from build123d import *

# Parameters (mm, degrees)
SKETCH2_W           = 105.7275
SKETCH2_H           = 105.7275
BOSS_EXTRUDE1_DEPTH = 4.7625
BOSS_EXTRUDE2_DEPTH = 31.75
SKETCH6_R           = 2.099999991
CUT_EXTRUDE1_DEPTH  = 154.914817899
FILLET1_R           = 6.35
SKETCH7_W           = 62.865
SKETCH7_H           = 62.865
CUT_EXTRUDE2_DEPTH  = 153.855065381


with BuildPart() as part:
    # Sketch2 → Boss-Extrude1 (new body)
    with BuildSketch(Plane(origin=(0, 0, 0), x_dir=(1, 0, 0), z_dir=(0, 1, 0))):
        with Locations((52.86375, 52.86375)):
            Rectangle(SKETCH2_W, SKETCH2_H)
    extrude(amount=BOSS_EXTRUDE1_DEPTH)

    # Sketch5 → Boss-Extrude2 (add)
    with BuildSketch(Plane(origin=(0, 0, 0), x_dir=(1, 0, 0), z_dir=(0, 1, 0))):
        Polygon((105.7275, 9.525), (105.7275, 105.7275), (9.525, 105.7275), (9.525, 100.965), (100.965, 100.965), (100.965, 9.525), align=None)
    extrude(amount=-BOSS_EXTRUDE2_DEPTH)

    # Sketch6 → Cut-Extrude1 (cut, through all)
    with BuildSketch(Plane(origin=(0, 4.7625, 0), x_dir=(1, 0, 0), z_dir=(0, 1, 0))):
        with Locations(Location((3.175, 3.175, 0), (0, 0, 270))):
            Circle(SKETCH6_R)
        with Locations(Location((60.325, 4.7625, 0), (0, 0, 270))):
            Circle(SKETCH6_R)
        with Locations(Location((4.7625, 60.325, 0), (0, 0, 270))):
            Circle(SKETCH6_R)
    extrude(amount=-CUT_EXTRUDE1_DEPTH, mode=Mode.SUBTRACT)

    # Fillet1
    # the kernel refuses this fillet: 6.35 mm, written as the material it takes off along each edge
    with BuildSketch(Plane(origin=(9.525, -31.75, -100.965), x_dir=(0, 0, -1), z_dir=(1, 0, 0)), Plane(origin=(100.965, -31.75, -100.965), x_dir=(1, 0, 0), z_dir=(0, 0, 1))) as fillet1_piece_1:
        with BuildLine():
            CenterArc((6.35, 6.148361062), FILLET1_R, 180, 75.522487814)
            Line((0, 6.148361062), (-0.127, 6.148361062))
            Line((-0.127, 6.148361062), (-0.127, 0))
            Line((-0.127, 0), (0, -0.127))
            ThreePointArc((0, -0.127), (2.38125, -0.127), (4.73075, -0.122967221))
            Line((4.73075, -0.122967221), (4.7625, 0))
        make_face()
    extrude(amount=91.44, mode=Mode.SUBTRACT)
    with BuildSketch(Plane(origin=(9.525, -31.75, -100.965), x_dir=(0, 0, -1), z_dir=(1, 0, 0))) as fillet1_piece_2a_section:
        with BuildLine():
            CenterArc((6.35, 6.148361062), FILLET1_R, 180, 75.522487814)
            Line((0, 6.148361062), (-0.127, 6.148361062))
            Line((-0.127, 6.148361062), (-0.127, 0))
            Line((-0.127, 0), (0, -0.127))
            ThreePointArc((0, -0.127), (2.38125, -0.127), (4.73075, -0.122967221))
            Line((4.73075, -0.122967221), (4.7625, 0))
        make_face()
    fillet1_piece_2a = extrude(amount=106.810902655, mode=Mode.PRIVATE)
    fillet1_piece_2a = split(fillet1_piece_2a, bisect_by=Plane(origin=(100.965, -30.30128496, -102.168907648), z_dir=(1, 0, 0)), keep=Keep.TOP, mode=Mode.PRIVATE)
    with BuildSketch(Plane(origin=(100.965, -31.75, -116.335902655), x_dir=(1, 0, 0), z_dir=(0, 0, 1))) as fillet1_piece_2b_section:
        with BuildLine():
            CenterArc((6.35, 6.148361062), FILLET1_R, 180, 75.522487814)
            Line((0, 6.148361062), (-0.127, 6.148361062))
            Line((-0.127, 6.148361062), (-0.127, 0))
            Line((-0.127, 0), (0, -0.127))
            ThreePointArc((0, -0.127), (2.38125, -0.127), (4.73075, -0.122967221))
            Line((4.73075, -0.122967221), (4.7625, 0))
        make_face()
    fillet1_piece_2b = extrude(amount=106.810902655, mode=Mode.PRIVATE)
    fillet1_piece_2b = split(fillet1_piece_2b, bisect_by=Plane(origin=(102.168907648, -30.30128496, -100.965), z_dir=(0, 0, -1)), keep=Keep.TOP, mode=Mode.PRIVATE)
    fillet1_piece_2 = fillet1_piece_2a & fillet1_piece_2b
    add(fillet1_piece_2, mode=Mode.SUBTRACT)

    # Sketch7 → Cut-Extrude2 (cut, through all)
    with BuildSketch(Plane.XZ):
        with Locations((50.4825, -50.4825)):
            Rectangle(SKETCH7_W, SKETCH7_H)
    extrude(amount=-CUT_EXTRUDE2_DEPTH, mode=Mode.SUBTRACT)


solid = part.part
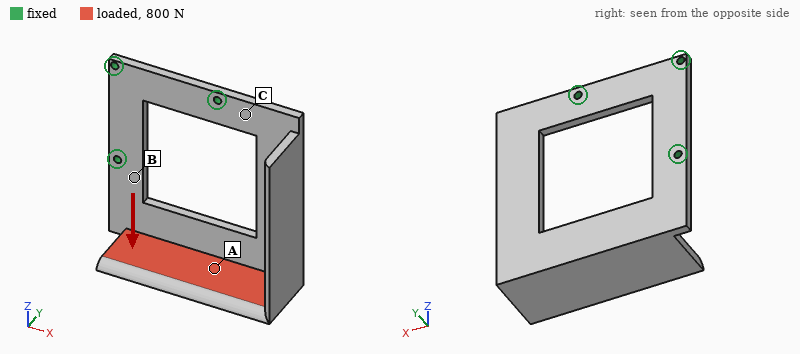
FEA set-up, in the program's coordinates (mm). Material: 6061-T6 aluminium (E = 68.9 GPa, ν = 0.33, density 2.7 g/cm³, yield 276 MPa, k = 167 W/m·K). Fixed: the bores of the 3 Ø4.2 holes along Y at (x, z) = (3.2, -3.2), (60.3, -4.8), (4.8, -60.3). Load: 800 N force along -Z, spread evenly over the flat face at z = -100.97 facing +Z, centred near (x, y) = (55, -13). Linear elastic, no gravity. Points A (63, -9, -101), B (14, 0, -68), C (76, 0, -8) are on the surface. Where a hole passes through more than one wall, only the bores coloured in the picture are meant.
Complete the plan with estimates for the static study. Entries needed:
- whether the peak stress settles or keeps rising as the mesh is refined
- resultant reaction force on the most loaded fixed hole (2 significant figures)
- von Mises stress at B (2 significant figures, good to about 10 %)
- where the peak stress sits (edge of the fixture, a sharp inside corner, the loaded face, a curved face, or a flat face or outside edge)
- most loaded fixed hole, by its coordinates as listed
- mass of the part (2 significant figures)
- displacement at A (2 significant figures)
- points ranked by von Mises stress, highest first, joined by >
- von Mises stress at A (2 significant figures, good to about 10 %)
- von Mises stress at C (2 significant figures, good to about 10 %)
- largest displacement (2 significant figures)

keeps rising
580 N
80 MPa
edge of the fixture
(60.3, -4.8)
170 g
0.78 mm
B > C > A
15 MPa
66 MPa
1.2 mm
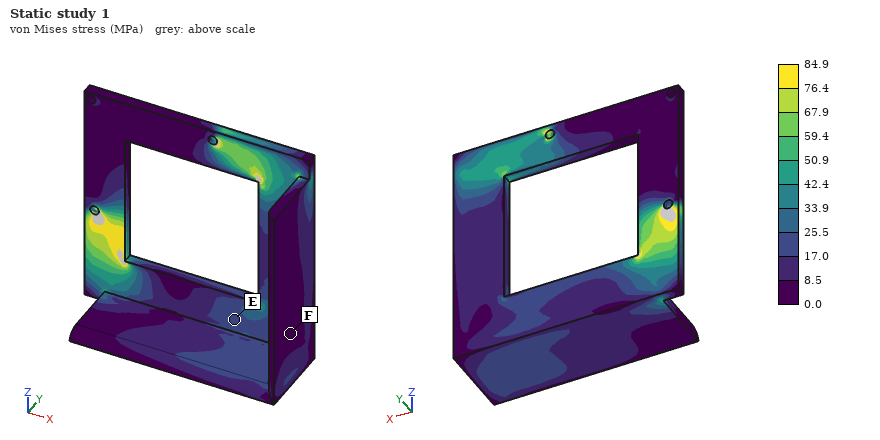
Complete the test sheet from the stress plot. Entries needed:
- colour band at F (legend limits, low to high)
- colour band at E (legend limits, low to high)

0.0 to 8.5 MPa
17.0 to 25.5 MPa
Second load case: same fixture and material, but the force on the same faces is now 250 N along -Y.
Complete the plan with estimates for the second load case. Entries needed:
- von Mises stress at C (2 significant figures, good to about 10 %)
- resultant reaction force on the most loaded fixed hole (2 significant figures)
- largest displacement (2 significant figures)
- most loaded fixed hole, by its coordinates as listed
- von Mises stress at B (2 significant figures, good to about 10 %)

79 MPa
230 N
1.7 mm
(4.8, -60.3)
97 MPa
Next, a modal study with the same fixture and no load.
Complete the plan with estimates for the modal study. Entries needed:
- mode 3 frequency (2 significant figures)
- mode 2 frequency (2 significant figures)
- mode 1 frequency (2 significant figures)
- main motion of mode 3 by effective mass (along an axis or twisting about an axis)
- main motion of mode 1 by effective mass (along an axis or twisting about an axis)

1300 Hz
800 Hz
220 Hz
along Y
along Y
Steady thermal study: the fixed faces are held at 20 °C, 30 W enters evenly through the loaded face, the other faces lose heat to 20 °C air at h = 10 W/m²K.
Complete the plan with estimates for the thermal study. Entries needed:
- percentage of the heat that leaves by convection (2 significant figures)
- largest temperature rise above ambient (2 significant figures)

24 %
47 K
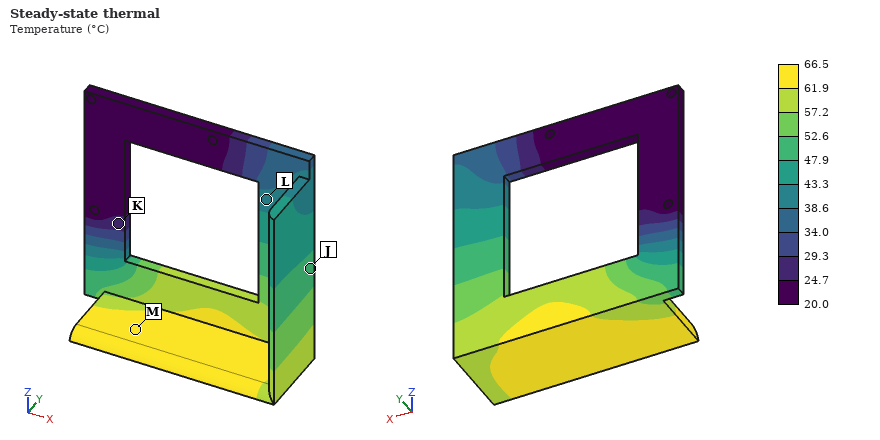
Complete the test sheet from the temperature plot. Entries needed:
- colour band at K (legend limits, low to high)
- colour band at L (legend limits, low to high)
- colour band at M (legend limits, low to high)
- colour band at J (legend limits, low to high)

24.7 to 29.3 °C
38.6 to 43.3 °C
61.9 to 66.5 °C
47.9 to 52.6 °C
